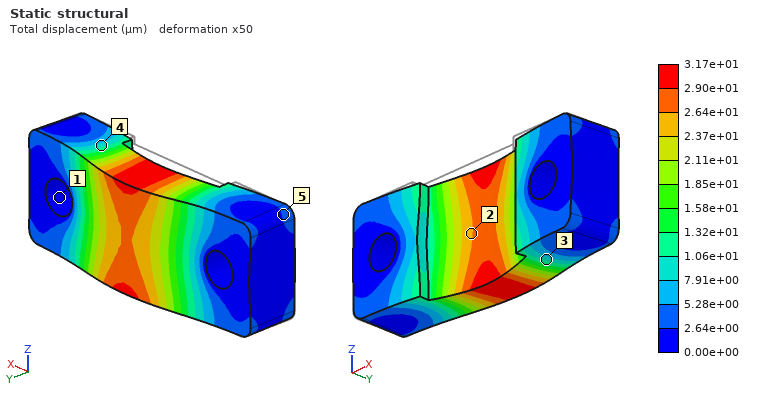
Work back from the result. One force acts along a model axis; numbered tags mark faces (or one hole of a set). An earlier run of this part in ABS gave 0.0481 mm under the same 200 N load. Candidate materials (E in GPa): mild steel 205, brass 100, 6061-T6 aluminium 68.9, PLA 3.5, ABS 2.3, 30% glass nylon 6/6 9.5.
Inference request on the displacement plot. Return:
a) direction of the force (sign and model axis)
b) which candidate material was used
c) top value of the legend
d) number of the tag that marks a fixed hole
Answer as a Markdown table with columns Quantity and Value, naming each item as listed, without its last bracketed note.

| Quantity | Value |
|---|---|
| direction of the force | +Y |
| which candidate material was used | PLA |
| top value of the legend | 3.17e+01 µm |
| number of the tag that marks a fixed hole | 1 |
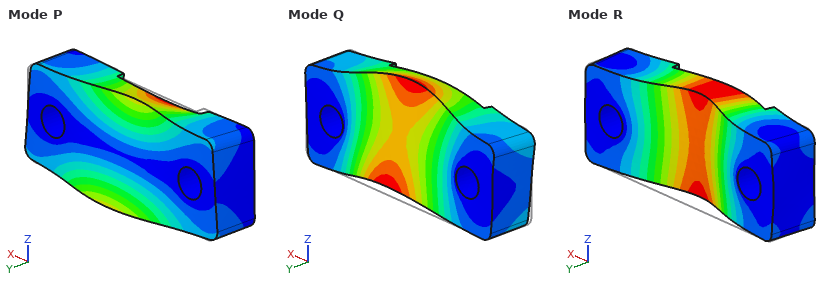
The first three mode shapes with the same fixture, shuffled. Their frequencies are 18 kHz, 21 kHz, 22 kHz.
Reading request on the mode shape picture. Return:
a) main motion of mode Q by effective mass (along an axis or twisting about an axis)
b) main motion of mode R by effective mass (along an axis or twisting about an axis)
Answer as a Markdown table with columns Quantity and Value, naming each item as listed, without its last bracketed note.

| Quantity | Value |
|---|---|
| main motion of mode Q by effective mass | along Z |
| main motion of mode R by effective mass | along Y |
